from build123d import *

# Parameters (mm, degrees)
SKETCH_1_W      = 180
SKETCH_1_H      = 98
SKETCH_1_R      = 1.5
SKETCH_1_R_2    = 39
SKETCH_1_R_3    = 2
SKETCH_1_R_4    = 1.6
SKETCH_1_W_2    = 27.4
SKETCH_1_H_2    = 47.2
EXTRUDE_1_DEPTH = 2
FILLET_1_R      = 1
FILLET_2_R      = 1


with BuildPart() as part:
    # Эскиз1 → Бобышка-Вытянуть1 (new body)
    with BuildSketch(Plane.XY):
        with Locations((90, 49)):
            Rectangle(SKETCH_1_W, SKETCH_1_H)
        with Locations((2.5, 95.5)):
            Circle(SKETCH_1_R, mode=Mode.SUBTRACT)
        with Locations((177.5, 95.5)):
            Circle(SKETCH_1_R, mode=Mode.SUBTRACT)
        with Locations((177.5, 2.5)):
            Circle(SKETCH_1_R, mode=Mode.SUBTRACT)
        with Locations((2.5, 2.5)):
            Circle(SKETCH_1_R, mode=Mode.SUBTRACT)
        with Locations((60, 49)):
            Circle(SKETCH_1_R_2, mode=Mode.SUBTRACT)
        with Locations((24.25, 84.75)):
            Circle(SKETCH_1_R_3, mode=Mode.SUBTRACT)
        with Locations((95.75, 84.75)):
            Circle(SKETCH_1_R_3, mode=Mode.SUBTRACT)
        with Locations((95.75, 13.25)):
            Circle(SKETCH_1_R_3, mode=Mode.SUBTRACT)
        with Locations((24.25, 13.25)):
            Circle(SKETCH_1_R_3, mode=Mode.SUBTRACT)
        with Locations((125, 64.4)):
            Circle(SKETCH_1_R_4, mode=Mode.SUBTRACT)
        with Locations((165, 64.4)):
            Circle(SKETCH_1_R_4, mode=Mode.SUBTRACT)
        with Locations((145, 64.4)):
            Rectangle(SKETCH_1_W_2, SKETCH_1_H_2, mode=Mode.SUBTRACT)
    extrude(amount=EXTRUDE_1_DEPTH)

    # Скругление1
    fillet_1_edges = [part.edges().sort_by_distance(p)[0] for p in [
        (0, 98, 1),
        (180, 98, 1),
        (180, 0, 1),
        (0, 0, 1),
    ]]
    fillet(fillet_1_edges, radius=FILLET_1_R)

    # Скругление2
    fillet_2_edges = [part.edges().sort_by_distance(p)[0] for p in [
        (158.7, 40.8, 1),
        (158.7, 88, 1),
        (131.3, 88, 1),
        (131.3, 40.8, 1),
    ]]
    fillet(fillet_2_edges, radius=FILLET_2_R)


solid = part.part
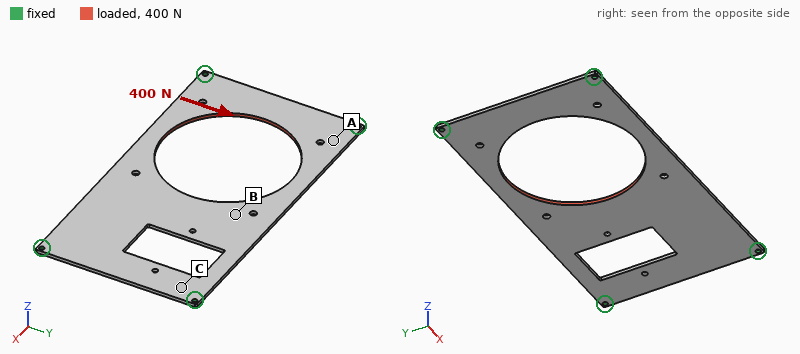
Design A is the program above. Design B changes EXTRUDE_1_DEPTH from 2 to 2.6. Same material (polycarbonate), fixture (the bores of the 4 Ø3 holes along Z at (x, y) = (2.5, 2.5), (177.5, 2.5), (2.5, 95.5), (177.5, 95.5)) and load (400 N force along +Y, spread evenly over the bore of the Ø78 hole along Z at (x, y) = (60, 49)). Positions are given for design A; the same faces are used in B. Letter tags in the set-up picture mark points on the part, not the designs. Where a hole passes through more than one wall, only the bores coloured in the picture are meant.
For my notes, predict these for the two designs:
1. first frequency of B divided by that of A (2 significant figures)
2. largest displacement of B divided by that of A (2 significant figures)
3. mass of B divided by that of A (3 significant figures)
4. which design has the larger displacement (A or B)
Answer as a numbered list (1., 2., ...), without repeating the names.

1. 1.3
2. 0.77
3. 1.30
4. A
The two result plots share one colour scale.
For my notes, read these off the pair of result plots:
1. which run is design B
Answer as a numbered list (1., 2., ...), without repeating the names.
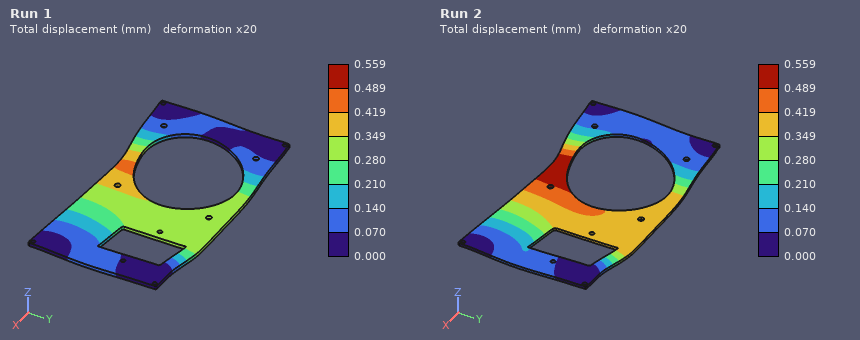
1. Run 1
